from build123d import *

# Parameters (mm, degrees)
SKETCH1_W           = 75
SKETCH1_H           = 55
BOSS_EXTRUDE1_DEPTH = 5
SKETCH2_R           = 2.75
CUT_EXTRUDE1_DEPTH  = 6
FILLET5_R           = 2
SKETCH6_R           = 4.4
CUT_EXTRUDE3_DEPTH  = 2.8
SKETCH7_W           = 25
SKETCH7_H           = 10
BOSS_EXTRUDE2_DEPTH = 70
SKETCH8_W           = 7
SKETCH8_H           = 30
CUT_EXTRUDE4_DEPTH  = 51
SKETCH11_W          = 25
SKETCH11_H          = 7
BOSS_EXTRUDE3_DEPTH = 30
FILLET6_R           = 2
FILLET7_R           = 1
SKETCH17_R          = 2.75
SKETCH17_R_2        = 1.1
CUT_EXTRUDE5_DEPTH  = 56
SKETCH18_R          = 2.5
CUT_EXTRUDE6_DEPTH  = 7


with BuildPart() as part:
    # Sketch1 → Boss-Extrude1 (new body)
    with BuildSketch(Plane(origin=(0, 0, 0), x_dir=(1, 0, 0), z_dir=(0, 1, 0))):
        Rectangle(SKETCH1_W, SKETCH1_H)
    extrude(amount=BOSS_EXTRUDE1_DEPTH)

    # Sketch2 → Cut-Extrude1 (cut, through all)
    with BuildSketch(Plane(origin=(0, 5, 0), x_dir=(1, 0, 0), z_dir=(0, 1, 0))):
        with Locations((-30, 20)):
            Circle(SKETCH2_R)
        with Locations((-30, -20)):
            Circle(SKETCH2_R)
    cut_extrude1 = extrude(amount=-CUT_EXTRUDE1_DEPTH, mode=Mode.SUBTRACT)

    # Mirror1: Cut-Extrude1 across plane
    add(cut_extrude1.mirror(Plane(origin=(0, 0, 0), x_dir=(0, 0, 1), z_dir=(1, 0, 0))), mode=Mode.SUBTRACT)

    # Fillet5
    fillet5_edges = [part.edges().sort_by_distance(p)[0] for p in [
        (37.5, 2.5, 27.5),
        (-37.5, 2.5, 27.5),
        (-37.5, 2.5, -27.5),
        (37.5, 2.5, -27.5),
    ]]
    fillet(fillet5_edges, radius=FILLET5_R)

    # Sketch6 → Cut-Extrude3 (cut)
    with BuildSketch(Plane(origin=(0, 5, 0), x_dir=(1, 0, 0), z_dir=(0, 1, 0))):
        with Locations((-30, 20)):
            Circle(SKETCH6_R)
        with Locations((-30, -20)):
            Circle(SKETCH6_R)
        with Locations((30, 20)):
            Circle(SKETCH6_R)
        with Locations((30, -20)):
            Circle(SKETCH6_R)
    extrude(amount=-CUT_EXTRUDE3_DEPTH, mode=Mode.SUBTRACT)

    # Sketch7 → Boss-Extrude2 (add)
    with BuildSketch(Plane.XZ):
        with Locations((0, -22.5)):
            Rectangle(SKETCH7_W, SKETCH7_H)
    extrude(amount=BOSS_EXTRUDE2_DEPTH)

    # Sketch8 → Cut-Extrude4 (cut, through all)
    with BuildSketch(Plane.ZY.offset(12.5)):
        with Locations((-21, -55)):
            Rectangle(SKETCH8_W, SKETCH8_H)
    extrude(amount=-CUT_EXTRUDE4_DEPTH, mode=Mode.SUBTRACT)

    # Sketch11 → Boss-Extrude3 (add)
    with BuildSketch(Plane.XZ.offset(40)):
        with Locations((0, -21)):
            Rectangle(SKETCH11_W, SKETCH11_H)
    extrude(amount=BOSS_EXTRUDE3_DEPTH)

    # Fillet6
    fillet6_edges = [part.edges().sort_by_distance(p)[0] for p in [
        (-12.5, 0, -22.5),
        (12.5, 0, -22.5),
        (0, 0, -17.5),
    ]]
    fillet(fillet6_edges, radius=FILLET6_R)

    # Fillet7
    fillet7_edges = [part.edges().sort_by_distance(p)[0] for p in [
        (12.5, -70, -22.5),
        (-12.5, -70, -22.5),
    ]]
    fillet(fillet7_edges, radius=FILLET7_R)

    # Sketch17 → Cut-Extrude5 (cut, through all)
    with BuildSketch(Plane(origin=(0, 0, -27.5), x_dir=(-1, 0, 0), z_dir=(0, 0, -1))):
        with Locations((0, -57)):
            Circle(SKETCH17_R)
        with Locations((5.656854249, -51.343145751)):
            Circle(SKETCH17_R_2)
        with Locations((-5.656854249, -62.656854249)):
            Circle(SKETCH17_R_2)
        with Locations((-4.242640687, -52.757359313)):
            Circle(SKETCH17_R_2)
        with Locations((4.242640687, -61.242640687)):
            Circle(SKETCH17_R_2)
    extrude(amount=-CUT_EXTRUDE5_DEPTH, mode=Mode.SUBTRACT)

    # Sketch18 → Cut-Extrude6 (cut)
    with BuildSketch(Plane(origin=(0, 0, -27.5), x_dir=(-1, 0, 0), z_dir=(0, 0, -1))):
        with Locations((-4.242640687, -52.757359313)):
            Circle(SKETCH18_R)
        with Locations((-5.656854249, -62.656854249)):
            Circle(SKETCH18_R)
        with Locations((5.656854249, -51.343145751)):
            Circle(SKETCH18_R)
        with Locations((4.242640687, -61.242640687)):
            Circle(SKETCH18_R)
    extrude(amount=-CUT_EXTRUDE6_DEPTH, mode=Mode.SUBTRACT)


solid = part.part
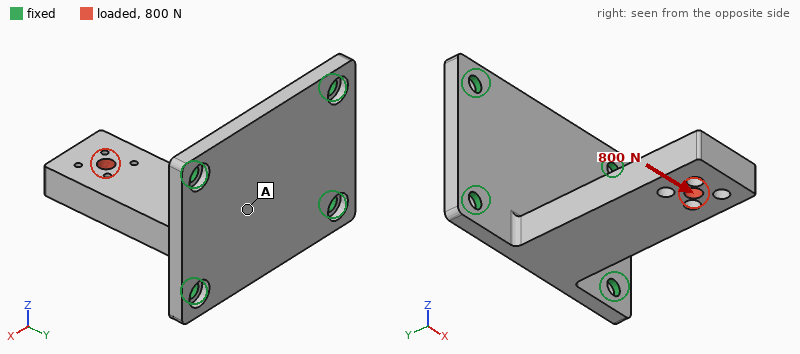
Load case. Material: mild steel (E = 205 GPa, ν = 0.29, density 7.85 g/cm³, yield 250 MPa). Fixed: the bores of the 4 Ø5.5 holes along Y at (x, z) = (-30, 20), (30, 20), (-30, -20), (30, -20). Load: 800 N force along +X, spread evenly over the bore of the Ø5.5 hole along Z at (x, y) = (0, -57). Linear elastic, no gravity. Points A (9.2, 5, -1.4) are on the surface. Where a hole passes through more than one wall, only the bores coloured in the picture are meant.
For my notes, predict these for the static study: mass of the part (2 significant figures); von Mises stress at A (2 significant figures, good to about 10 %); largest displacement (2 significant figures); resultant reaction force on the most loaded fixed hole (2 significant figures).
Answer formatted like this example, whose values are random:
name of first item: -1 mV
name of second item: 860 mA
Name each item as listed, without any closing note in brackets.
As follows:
mass of the part: 290 g
von Mises stress at A: 23 MPa
largest displacement: 0.12 mm
resultant reaction force on the most loaded fixed hole: 970 N
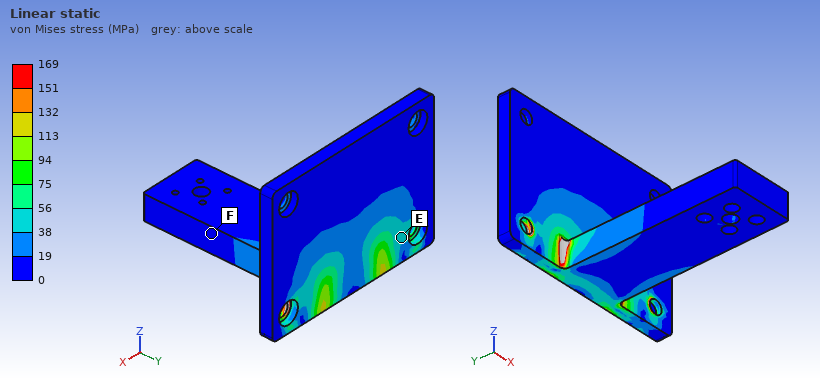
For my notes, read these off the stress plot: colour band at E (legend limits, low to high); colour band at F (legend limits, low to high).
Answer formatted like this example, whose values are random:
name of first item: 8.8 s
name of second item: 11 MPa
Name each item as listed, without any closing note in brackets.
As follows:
colour band at E: 38 to 56 MPa
colour band at F: 0 to 19 MPa
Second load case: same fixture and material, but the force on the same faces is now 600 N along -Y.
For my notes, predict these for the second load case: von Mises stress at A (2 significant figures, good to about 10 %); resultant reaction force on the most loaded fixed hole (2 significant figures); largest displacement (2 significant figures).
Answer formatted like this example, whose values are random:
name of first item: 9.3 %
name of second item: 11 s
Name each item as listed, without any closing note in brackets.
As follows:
von Mises stress at A: 7.2 MPa
resultant reaction force on the most loaded fixed hole: 370 N
largest displacement: 29 µm
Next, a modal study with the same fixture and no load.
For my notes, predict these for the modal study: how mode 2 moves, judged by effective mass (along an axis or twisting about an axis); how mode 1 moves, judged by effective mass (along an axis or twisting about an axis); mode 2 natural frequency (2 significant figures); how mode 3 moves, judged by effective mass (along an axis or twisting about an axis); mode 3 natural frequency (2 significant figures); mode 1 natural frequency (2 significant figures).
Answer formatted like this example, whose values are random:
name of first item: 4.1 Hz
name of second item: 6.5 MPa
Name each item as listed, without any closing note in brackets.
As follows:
how mode 2 moves, judged by effective mass: along X
how mode 1 moves, judged by effective mass: along Z
mode 2 natural frequency: 1800 Hz
how mode 3 moves, judged by effective mass: along Y
mode 3 natural frequency: 3400 Hz
mode 1 natural frequency: 900 Hz
